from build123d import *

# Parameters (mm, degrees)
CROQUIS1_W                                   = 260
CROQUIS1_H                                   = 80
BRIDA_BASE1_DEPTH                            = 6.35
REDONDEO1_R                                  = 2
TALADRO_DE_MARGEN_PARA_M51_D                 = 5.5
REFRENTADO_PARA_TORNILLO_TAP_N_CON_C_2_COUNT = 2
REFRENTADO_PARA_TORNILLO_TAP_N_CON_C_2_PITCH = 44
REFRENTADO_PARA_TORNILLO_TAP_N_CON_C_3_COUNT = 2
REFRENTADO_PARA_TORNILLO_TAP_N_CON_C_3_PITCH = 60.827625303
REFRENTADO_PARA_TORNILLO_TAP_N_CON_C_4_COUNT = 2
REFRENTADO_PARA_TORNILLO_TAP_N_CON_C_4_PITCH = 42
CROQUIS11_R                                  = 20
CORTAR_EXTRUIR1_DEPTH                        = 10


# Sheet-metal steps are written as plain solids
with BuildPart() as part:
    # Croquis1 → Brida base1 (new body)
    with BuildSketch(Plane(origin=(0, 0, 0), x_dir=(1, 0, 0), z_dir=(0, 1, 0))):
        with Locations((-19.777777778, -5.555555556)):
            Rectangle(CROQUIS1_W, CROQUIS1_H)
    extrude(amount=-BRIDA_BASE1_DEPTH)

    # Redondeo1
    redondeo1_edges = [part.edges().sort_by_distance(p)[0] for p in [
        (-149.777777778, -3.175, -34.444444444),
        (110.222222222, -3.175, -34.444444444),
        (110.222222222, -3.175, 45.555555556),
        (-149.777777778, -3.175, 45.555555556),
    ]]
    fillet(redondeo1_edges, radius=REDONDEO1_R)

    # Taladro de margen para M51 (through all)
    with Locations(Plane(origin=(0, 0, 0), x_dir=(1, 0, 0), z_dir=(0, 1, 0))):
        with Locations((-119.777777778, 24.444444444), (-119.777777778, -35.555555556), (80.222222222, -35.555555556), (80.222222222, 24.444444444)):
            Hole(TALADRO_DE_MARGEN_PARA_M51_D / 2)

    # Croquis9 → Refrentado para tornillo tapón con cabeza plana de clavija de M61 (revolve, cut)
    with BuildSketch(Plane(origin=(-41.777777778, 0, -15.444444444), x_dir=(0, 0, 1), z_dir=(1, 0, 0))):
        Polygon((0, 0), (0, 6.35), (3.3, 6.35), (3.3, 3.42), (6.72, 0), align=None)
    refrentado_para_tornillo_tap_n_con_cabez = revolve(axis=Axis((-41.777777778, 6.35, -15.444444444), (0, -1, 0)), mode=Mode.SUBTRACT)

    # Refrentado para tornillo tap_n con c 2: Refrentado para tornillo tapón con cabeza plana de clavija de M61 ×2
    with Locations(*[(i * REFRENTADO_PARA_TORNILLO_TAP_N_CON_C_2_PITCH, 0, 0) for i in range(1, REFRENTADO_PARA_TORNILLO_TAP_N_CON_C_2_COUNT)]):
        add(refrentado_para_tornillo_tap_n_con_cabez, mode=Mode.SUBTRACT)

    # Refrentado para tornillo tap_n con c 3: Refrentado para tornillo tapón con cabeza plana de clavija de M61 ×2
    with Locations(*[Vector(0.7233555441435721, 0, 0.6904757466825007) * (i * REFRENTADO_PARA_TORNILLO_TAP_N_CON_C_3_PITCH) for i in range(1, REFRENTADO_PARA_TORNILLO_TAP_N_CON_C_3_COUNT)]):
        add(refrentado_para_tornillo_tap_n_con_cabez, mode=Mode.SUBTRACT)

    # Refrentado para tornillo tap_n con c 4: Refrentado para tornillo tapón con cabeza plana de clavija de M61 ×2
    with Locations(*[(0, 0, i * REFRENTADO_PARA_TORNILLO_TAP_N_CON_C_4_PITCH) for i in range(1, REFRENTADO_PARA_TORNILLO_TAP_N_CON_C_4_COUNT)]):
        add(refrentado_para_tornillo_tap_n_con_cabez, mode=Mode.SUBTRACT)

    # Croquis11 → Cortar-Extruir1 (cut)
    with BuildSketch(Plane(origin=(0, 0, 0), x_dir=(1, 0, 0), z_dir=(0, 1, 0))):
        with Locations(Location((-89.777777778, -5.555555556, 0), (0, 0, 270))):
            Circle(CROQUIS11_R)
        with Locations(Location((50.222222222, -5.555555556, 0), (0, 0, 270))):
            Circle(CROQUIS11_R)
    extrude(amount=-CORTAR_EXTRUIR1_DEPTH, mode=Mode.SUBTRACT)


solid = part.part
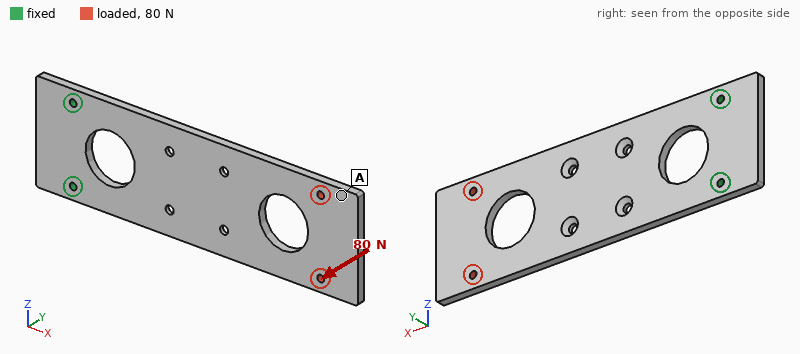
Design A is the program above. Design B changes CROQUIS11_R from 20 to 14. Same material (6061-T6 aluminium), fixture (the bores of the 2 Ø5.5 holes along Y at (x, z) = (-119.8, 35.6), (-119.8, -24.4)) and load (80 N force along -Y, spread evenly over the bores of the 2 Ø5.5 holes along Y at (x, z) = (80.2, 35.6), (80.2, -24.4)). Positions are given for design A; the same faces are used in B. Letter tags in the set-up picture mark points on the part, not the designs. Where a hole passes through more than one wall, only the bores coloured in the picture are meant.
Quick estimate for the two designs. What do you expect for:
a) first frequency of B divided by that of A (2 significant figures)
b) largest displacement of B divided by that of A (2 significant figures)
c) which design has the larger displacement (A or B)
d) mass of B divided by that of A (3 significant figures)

1.1
0.85
A
1.07
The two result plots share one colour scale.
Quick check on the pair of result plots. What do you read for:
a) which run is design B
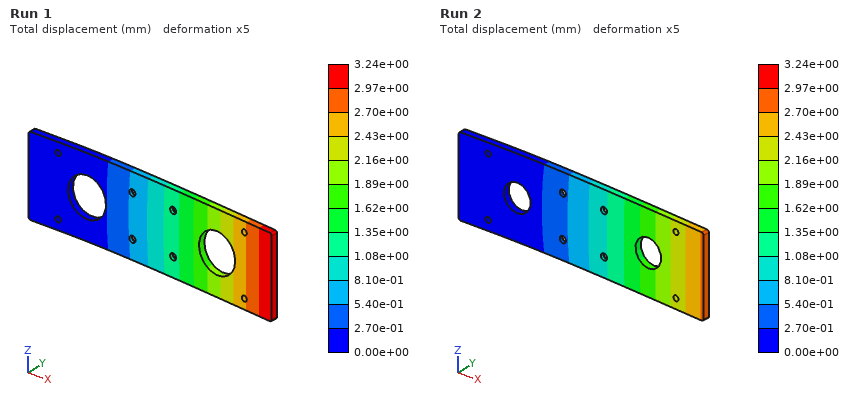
Run 2
